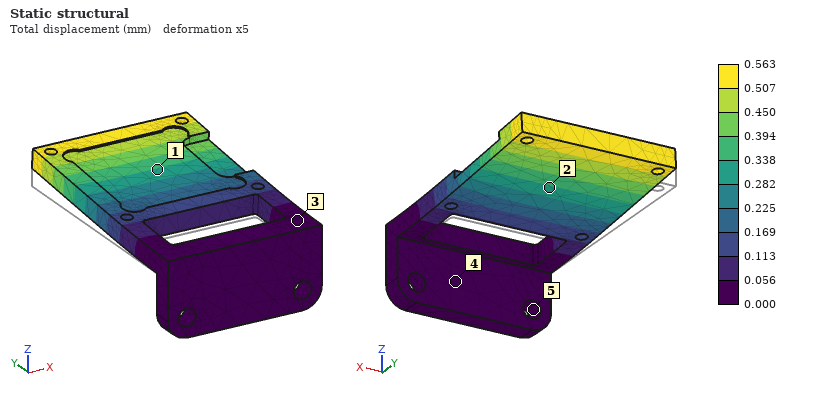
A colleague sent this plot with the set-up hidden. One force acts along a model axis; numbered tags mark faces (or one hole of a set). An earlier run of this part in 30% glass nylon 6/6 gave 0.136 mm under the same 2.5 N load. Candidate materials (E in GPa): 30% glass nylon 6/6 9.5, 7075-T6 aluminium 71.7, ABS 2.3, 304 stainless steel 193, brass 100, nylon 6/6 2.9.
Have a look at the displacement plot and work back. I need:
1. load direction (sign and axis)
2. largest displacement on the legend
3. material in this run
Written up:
+Z
0.563 mm
ABS
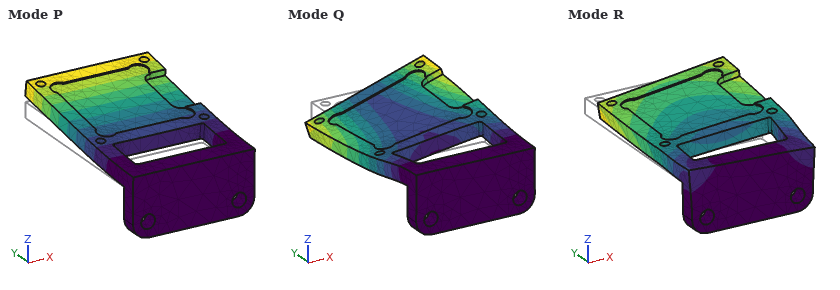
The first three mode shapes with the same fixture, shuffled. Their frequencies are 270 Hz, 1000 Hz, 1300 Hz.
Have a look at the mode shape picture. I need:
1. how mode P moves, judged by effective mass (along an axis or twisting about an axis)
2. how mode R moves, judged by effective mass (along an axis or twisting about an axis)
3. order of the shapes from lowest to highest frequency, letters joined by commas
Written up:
along Z
along X
P, R, Q
